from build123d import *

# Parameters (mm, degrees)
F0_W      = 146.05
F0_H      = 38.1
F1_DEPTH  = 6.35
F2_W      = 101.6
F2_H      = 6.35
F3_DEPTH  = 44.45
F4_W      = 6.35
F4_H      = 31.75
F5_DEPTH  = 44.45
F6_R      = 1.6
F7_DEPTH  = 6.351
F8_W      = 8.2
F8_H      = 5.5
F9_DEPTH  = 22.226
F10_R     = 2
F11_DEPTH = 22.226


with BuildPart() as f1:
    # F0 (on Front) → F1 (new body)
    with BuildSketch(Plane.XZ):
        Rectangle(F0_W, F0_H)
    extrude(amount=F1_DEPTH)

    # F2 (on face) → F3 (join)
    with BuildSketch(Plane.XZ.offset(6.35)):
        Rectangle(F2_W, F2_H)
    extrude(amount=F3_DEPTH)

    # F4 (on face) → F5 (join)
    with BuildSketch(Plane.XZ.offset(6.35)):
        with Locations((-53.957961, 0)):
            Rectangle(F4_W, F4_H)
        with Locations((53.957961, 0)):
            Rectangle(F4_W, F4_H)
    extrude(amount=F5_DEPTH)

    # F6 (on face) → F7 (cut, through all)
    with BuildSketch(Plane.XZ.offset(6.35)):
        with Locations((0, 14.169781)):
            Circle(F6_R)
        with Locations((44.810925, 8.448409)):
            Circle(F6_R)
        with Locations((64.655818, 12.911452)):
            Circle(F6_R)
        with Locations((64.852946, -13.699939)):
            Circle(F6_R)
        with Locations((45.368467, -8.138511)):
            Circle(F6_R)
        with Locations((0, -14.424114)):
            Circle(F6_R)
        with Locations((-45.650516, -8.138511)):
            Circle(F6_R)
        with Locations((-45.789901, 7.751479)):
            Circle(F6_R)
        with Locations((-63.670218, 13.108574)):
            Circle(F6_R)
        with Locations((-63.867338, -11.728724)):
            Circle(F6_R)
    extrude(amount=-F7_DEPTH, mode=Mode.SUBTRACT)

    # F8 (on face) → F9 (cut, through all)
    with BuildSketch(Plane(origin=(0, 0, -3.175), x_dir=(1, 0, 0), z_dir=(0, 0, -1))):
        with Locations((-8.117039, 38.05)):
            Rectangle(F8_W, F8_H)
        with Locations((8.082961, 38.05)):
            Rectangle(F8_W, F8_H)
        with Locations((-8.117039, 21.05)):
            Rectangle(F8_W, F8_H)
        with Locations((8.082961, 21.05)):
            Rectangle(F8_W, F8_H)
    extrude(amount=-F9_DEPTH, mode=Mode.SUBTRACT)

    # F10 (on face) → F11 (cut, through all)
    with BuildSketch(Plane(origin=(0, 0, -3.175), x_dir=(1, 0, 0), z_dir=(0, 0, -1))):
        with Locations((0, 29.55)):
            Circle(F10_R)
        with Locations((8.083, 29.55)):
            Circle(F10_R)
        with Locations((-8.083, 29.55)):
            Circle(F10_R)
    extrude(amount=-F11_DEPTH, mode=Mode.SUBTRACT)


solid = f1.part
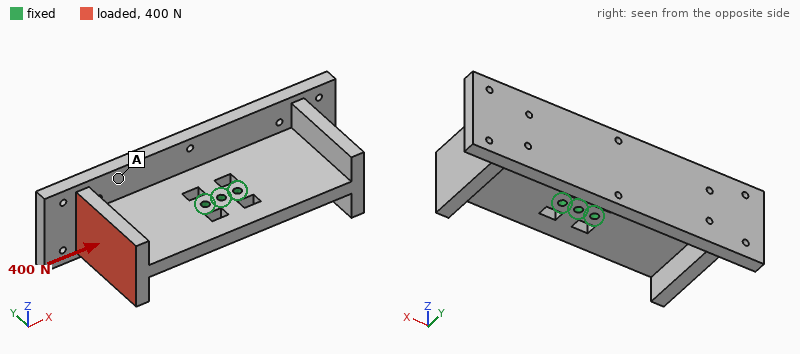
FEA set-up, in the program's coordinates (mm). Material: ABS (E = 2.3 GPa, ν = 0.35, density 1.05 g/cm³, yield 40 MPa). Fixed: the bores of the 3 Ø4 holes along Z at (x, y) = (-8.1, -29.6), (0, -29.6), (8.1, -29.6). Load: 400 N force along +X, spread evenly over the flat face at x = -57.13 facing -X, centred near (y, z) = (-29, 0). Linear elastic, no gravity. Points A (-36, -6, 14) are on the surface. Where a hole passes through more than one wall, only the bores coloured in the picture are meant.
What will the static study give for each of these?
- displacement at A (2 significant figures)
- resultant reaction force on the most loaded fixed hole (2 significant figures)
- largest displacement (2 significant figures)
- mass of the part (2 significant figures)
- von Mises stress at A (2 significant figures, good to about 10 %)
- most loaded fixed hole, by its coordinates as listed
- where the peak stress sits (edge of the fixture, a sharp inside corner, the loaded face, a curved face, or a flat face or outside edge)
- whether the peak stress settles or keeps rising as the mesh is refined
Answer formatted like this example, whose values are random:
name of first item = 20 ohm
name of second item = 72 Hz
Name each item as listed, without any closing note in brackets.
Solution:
displacement at A = 26 µm
resultant reaction force on the most loaded fixed hole = 250 N
largest displacement = 73 µm
mass of the part = 84 g
von Mises stress at A = 0.41 MPa
most loaded fixed hole, by its coordinates as listed = (-8.1, -29.6)
where the peak stress sits = edge of the fixture
whether the peak stress settles or keeps rising as the mesh is refined = keeps rising
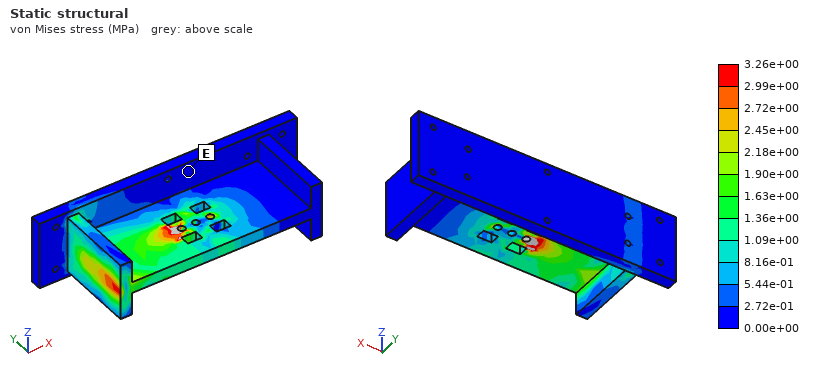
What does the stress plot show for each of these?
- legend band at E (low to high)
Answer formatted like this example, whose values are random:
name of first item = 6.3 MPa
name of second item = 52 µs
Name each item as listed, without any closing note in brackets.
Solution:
legend band at E = 0.00e+00 to 2.72e-01 MPa
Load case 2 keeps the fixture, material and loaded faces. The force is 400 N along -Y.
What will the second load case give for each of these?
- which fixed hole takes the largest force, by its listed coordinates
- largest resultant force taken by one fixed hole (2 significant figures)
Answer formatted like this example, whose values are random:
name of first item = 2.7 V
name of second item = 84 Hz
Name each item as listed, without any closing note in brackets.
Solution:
which fixed hole takes the largest force, by its listed coordinates = (-8.1, -29.6)
largest resultant force taken by one fixed hole = 1.2 kN
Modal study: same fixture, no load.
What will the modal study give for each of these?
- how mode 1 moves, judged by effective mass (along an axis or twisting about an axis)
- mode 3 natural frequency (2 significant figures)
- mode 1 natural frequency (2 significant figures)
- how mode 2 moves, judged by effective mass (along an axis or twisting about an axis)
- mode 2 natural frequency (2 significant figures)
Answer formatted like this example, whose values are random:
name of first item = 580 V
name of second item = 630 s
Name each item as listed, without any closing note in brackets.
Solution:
how mode 1 moves, judged by effective mass = twisting about Y
mode 3 natural frequency = 510 Hz
mode 1 natural frequency = 260 Hz
how mode 2 moves, judged by effective mass = along Z
mode 2 natural frequency = 380 Hz
